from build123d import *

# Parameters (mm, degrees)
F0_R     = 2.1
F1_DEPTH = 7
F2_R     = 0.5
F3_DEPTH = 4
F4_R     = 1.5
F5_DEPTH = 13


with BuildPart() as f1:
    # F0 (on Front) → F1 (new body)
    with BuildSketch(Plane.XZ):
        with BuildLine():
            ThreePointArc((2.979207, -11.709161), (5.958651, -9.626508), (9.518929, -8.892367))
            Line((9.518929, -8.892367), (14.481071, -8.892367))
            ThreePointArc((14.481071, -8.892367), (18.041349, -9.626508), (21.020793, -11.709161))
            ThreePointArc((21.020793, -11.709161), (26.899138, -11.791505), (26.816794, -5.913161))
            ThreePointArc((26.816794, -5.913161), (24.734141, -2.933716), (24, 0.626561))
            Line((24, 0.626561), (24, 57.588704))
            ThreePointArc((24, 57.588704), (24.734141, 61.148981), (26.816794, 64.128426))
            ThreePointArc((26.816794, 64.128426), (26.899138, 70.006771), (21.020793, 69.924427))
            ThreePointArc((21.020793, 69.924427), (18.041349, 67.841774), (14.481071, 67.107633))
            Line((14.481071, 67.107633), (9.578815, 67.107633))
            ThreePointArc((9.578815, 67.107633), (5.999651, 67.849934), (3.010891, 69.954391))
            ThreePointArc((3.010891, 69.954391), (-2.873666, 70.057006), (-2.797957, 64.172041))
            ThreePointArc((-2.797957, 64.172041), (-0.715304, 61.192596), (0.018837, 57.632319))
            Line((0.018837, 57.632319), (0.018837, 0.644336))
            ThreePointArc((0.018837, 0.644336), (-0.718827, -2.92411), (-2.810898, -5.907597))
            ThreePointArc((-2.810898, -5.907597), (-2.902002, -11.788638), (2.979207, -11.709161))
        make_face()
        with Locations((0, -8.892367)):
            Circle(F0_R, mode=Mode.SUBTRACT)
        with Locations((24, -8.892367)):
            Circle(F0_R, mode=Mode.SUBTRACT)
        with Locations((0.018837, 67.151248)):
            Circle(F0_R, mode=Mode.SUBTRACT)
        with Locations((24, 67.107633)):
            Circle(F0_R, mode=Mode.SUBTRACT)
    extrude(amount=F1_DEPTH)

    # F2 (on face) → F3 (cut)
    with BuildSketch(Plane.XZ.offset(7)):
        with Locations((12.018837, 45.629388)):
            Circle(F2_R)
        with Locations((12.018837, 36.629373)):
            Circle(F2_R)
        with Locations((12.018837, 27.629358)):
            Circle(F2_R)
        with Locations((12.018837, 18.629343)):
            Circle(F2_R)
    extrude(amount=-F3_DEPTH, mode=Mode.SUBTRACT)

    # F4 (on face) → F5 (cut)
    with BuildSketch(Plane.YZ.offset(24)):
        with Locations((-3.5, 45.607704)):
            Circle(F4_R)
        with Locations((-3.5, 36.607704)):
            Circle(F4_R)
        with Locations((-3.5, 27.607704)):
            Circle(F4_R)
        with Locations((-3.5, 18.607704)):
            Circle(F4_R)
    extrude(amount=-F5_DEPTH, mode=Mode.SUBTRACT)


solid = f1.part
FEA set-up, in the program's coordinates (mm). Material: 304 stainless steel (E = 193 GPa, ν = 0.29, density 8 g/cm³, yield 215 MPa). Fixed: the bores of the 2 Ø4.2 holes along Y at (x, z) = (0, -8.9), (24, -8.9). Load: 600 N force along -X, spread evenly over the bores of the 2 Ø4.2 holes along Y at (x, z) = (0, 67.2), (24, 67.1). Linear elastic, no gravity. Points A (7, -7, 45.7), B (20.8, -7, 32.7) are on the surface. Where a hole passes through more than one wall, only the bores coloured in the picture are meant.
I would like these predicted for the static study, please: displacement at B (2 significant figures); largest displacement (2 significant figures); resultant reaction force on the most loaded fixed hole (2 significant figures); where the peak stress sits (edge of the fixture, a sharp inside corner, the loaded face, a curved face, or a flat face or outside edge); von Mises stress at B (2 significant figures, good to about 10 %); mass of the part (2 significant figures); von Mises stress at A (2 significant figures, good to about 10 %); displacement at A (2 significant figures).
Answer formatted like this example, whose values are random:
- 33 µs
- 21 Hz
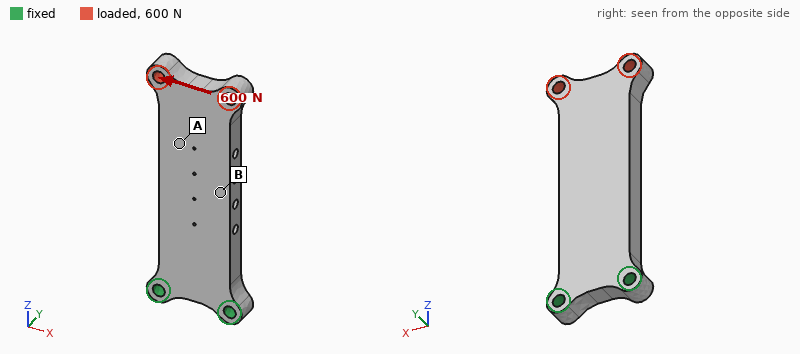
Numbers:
- 23 µm
- 67 µm
- 2.0 kN
- a curved face
- 32 MPa
- 110 g
- 12 MPa
- 35 µm
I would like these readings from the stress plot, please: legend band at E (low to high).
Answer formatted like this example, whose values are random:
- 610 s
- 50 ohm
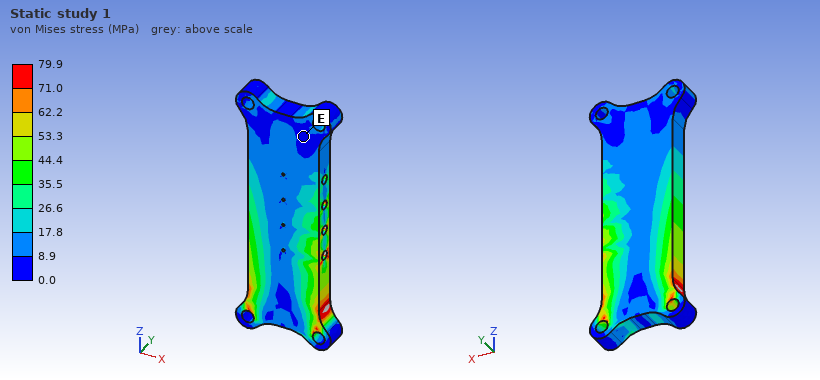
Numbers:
- 0.0 to 8.9 MPa
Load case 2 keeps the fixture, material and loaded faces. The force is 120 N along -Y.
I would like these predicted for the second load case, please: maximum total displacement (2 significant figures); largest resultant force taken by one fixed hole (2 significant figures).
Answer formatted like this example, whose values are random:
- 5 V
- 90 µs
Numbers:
- 0.16 mm
- 60 N
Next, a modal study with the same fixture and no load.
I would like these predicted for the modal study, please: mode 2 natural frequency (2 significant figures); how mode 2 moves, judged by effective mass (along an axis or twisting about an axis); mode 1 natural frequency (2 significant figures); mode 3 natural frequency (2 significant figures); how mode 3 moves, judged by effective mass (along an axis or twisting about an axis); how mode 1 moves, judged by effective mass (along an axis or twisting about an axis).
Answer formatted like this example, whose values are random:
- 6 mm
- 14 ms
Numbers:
- 3000 Hz
- along X
- 860 Hz
- 4900 Hz
- twisting about Z
- along Y
